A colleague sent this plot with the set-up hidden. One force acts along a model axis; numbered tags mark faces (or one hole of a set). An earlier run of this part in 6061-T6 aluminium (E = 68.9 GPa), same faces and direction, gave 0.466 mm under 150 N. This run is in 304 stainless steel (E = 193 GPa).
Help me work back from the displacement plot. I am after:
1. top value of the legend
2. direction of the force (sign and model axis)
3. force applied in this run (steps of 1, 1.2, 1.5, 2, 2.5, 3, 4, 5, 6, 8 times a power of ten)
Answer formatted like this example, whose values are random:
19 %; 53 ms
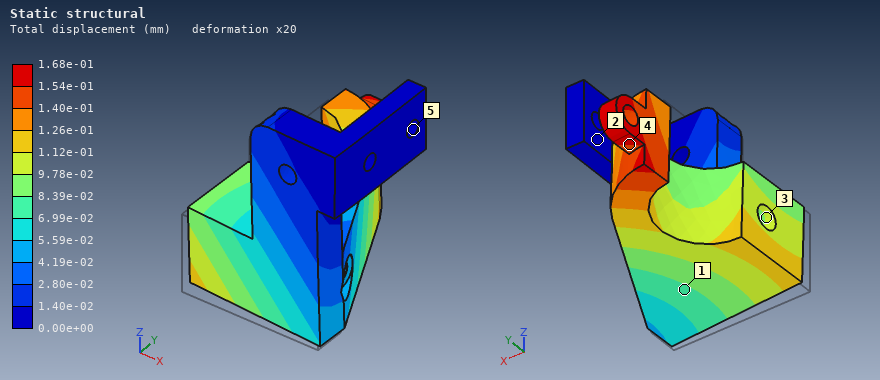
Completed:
1.68e-01 mm; +Y; 150 N
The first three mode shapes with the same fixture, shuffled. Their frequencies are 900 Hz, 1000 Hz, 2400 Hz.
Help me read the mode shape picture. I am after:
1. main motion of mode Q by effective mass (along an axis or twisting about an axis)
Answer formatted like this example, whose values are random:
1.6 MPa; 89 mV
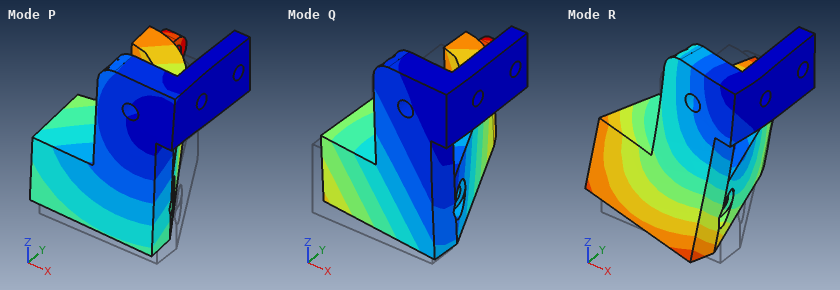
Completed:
along Y
